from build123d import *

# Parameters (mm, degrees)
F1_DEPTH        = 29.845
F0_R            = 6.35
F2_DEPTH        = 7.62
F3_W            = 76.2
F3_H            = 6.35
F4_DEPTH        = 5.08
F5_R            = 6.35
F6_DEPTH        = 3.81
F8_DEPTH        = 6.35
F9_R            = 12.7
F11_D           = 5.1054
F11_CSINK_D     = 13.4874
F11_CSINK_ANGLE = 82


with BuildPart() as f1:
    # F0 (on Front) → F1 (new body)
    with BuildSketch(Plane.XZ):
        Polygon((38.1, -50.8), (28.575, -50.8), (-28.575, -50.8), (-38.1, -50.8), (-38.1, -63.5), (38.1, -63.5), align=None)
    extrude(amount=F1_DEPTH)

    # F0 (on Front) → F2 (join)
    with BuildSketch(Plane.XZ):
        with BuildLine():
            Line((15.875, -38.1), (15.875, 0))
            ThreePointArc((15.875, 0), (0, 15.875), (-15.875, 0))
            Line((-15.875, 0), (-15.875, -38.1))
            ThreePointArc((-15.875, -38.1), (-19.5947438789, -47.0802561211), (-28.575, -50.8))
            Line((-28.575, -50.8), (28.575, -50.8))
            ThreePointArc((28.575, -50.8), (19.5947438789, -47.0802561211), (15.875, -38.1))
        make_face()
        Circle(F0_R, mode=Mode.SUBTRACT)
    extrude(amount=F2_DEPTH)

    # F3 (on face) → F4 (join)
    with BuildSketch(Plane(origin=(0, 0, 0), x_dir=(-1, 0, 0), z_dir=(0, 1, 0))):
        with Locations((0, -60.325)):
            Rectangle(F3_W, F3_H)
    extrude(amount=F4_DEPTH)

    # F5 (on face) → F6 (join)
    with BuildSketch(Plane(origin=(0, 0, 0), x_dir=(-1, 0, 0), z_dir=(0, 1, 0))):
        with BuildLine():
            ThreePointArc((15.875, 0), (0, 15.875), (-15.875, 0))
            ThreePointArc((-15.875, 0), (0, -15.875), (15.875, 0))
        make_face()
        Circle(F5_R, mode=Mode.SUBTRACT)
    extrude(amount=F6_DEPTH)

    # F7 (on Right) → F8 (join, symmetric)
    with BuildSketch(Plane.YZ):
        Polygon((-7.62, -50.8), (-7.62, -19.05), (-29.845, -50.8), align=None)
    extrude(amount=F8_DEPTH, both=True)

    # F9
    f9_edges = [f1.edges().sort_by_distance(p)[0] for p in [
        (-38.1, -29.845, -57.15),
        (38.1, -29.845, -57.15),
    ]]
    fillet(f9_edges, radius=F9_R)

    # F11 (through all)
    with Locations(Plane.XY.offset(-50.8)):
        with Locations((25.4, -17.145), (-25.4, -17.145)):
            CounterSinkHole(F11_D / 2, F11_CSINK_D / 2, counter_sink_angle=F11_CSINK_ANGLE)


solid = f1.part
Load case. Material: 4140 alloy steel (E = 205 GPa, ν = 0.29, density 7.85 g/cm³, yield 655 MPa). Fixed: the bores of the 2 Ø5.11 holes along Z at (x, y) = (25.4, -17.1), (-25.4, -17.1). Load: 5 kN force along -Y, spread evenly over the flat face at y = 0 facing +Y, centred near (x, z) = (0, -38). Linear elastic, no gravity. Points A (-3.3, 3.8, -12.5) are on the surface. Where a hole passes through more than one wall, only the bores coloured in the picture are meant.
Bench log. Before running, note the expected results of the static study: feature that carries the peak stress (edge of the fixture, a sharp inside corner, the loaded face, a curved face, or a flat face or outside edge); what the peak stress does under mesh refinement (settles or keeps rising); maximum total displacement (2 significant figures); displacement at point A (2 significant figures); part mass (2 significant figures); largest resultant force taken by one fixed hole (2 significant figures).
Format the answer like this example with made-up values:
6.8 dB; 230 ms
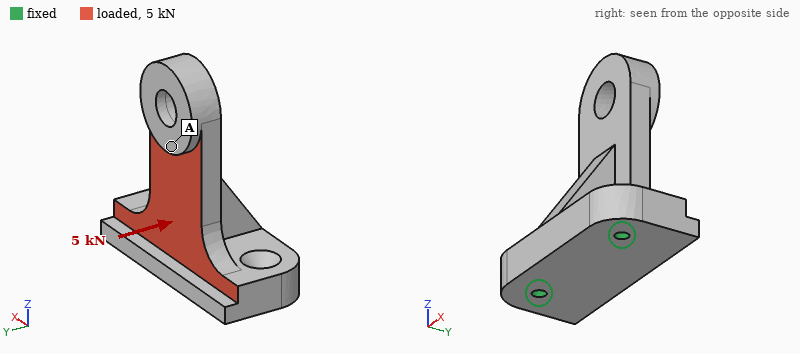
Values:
edge of the fixture; keeps rising; 0.12 mm; 0.078 mm; 400 g; 2.6 kN
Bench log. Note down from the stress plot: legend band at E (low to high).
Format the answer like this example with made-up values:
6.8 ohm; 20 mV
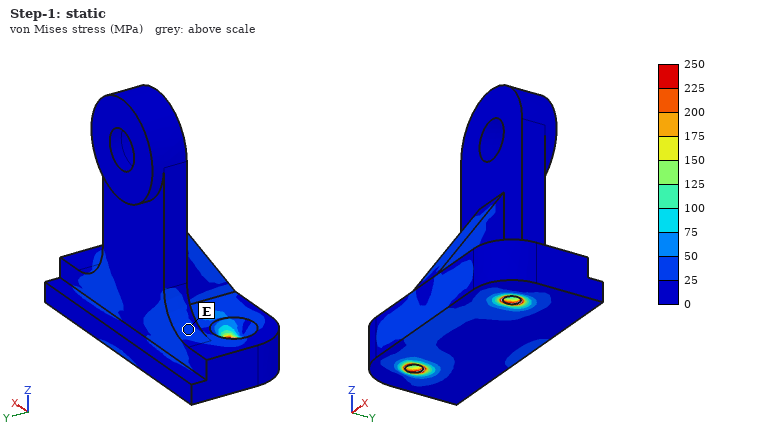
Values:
25 to 50 MPa
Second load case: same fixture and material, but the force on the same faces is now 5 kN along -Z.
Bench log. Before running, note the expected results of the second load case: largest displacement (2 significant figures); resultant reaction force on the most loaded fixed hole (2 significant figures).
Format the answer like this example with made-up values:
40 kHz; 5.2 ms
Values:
84 µm; 2.6 kN
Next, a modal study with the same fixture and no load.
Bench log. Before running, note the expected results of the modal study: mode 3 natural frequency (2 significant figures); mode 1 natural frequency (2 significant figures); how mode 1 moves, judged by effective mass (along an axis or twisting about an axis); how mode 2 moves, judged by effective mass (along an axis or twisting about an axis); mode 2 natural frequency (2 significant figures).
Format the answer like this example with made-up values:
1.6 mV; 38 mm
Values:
6400 Hz; 2000 Hz; along Y; along X; 4300 Hz
